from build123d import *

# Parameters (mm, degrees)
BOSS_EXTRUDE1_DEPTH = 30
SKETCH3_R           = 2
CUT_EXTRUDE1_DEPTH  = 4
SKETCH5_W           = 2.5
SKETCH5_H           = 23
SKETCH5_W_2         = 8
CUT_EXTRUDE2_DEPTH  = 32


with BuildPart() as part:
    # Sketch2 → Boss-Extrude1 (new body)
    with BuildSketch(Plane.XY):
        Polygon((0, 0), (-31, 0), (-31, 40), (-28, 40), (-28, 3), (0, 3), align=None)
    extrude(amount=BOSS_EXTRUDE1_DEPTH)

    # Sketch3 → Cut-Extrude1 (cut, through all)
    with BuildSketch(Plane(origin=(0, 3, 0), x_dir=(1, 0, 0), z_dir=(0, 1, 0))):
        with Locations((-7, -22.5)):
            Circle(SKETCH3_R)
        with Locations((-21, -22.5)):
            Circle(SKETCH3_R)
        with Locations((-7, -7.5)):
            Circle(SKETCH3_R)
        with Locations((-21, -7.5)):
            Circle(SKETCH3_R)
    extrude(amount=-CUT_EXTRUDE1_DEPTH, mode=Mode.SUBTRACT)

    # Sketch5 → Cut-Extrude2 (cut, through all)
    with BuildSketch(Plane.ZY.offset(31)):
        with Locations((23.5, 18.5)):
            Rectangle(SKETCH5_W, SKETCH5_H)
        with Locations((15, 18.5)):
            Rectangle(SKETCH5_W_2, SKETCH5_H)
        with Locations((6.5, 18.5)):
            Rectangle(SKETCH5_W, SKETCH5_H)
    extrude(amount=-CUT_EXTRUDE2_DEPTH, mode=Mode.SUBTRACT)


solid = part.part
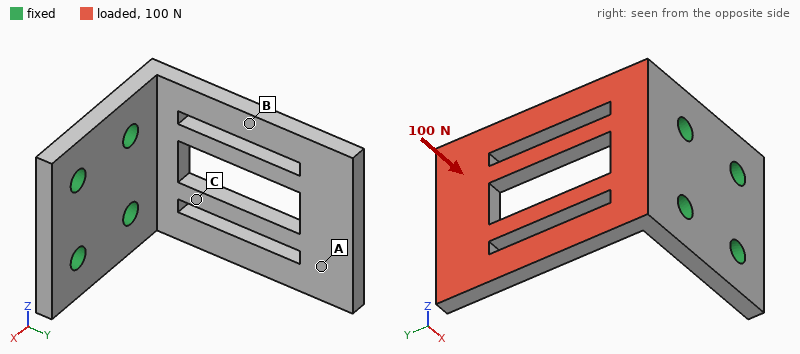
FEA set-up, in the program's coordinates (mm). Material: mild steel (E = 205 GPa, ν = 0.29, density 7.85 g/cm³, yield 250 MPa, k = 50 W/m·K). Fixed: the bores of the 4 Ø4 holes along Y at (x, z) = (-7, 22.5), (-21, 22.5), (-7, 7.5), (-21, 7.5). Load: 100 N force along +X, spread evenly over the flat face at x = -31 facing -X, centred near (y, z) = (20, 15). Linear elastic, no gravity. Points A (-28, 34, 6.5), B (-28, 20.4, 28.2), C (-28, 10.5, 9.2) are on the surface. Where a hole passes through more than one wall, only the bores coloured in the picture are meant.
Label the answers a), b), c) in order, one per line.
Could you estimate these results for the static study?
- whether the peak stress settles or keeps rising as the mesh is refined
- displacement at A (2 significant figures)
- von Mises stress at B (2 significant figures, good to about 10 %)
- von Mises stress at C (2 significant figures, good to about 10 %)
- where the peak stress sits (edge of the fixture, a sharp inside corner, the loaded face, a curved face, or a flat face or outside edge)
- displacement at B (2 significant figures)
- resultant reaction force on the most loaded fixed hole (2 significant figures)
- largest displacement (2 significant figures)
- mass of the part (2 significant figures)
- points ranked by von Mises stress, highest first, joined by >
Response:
a) keeps rising
b) 0.093 mm
c) 22 MPa
d) 51 MPa
e) edge of the fixture
f) 0.043 mm
g) 46 N
h) 0.12 mm
i) 40 g
j) C > B > A
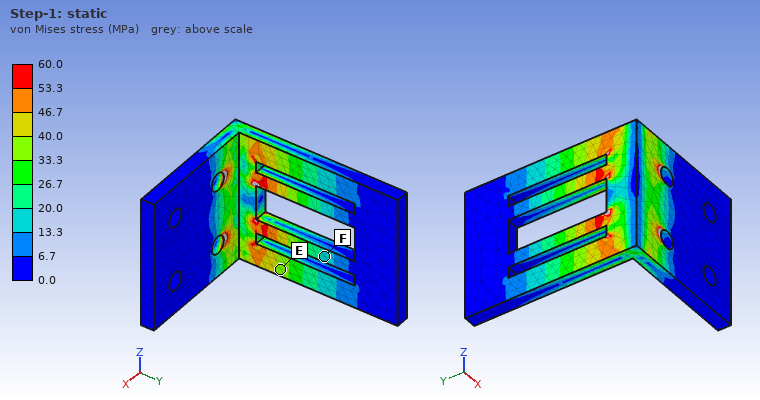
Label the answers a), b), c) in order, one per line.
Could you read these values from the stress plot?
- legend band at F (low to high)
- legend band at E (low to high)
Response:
a) 13.3 to 20.0 MPa
b) 33.3 to 40.0 MPa
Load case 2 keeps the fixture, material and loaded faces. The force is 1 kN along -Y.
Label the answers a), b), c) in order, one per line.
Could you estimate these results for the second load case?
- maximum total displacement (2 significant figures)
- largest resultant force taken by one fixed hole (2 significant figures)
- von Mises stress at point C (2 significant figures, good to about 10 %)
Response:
a) 0.19 mm
b) 550 N
c) 27 MPa
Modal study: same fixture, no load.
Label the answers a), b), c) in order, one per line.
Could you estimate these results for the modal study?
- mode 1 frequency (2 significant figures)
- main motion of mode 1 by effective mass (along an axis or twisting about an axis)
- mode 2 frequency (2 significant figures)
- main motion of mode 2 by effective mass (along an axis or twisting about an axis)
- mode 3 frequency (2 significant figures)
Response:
a) 1200 Hz
b) along X
c) 3000 Hz
d) along Z
e) 3700 Hz
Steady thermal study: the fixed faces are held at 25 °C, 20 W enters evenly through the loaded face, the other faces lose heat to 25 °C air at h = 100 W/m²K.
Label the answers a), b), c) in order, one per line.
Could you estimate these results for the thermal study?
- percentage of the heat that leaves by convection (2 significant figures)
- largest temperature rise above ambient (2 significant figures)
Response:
a) 48 %
b) 76 K
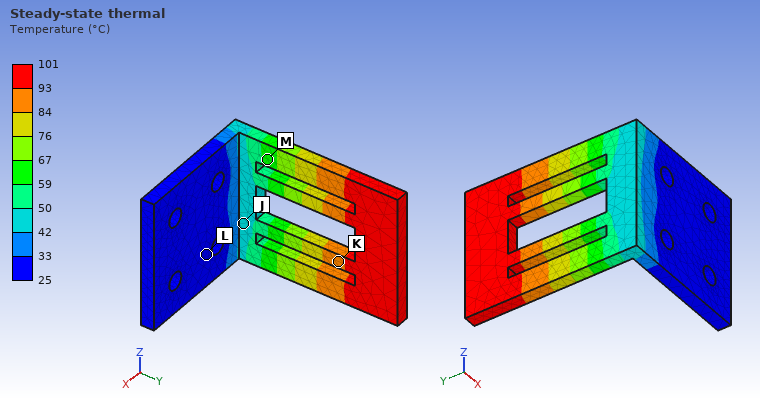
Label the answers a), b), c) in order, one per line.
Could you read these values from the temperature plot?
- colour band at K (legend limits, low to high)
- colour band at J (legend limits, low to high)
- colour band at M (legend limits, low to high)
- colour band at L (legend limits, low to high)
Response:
a) 84 to 93 °C
b) 42 to 50 °C
c) 59 to 67 °C
d) 25 to 33 °C
